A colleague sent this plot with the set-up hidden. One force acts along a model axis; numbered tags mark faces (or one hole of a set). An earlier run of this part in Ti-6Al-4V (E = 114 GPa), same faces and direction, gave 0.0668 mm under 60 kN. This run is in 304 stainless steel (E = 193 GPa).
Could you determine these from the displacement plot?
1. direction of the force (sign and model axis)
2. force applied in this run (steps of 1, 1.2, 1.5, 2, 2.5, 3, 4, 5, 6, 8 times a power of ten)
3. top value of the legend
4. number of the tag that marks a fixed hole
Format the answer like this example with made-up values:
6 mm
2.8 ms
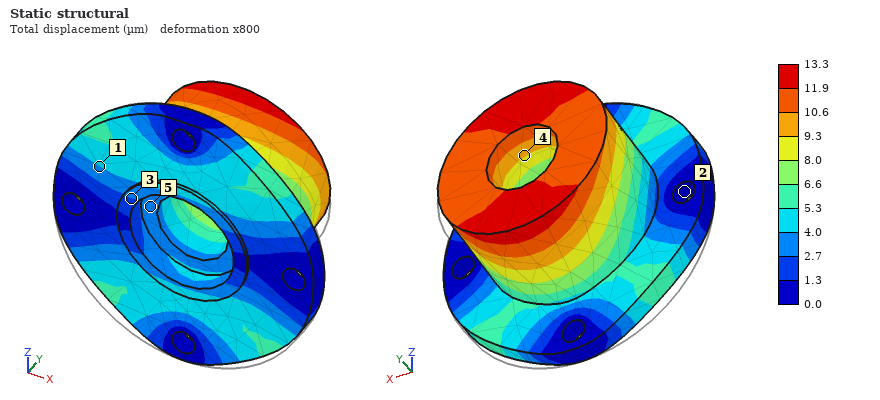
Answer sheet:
+Z
20 kN
13.3 µm
2
